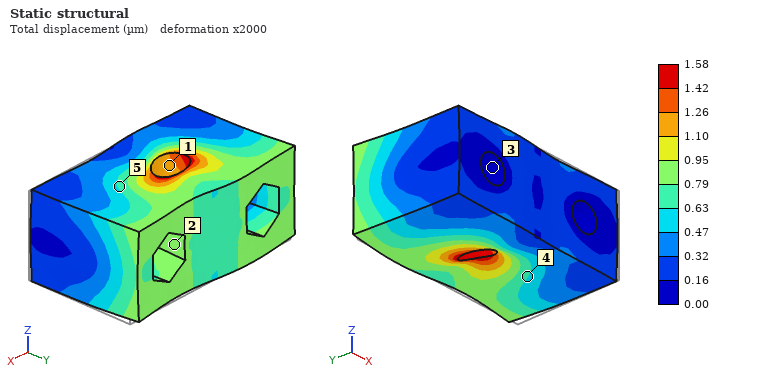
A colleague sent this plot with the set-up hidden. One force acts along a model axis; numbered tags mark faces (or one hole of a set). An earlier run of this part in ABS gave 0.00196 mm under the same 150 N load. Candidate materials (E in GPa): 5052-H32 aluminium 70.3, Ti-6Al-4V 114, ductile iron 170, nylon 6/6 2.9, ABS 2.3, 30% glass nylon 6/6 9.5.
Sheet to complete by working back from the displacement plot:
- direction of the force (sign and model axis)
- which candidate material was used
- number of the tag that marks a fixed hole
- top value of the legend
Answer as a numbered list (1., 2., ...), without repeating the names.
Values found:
1. -X
2. nylon 6/6
3. 3
4. 1.58 µm
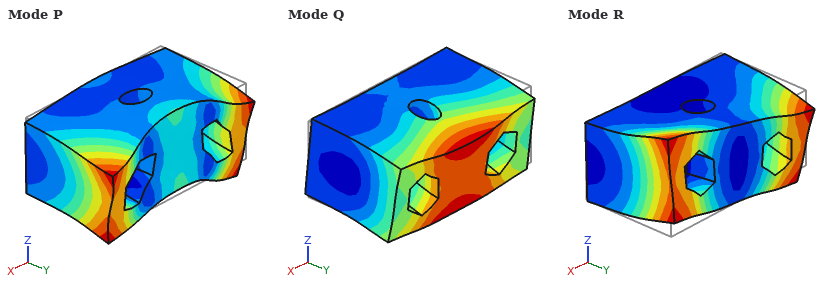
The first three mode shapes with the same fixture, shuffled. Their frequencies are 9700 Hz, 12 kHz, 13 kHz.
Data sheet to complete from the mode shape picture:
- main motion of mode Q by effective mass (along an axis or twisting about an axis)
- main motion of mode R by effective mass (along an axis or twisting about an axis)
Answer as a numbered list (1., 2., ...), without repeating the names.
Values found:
1. along Z
2. twisting about Y
